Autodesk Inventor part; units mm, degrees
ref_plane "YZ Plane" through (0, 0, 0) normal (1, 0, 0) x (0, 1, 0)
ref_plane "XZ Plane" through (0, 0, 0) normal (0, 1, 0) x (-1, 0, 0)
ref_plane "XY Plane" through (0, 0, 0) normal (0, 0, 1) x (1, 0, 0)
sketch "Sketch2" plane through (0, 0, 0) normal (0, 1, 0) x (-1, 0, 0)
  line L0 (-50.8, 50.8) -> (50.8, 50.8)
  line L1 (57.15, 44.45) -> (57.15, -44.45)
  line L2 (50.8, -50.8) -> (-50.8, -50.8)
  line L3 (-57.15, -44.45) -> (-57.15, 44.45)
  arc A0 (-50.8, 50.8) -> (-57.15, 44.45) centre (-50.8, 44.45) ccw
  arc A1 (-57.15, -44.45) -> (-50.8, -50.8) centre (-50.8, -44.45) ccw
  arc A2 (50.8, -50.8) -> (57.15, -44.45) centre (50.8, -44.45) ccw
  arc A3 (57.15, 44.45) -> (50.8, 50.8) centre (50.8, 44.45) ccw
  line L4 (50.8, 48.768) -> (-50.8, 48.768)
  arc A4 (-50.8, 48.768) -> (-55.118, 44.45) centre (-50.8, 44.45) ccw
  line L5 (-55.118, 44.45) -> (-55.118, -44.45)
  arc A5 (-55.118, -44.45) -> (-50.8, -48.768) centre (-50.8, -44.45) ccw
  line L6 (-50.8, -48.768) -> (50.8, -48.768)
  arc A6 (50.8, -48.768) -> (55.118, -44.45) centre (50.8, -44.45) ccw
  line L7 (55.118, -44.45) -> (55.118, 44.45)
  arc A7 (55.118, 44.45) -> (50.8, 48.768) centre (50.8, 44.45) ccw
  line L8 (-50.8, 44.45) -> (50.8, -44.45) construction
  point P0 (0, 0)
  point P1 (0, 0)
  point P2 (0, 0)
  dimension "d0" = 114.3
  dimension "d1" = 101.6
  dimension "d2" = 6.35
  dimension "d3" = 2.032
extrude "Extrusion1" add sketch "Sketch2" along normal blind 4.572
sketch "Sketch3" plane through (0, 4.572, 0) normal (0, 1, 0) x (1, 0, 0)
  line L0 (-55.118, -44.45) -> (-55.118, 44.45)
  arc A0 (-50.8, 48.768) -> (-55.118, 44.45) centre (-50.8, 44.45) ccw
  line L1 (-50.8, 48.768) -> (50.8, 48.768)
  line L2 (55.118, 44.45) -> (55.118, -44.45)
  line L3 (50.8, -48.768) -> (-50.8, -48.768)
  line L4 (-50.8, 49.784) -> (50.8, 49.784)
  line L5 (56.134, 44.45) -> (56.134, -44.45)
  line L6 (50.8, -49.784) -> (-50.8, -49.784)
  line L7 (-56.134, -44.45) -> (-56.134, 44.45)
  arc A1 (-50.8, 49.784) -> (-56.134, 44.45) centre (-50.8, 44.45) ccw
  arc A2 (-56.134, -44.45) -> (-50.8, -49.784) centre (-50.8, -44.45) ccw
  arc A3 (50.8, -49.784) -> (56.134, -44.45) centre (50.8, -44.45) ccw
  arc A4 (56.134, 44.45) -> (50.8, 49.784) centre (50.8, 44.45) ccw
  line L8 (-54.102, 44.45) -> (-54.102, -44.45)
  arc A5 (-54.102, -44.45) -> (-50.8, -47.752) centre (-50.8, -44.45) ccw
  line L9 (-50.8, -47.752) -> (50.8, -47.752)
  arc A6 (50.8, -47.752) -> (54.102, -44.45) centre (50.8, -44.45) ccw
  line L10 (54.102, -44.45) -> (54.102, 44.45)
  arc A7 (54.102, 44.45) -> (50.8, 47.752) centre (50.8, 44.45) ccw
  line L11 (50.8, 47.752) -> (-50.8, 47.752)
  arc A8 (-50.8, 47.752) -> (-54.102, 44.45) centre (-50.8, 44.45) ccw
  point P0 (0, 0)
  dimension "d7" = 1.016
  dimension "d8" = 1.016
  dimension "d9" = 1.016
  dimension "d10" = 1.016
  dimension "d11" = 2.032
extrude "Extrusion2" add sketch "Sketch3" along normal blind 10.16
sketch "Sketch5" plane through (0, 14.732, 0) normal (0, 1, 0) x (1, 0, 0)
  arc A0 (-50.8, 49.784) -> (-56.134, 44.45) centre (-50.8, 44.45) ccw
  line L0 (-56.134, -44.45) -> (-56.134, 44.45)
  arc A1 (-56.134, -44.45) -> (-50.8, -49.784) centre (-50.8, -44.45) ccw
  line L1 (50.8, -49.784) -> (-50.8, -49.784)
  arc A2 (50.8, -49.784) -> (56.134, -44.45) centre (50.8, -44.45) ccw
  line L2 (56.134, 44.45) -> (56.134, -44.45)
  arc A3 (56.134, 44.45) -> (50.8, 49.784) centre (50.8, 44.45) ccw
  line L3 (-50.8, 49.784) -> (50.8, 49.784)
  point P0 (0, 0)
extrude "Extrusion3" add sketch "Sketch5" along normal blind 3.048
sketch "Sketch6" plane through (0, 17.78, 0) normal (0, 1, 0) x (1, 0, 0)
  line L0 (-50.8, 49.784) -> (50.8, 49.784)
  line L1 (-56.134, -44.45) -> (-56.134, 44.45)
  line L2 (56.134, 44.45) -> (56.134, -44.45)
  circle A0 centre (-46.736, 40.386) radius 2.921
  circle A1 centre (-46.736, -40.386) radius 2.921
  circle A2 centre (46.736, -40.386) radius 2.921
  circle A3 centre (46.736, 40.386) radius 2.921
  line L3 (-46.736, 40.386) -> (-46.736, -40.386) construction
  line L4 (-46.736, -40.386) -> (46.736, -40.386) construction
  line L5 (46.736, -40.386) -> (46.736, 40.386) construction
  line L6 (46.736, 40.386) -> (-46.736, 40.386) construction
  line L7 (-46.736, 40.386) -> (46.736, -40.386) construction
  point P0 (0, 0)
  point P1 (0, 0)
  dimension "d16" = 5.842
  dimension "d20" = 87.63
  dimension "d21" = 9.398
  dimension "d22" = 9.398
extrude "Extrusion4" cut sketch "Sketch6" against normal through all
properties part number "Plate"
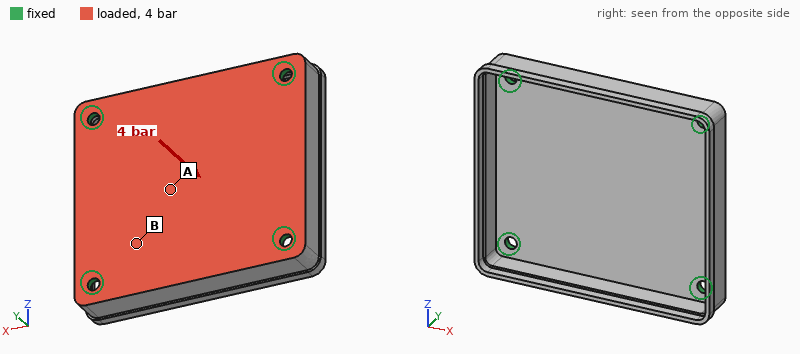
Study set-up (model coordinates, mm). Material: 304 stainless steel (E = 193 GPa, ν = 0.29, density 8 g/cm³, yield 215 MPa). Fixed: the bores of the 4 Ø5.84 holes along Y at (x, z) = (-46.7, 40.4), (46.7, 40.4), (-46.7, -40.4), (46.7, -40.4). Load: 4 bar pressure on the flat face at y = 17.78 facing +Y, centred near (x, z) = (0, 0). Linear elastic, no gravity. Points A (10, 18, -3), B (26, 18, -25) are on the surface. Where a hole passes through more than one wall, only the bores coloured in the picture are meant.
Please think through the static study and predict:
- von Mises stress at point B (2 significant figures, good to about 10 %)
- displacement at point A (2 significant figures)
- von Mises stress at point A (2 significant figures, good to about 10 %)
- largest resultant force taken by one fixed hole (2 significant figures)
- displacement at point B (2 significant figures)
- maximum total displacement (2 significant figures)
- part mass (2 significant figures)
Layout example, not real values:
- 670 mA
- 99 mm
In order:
- 44 MPa
- 0.23 mm
- 91 MPa
- 1.1 kN
- 0.11 mm
- 0.24 mm
- 370 g
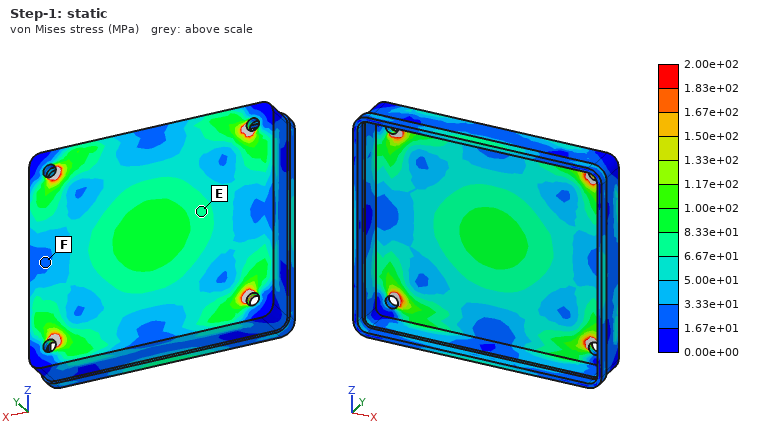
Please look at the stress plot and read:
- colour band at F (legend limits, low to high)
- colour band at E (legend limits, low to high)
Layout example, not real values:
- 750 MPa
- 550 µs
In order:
- 1.67e+01 to 3.33e+01 MPa
- 6.67e+01 to 8.33e+01 MPa
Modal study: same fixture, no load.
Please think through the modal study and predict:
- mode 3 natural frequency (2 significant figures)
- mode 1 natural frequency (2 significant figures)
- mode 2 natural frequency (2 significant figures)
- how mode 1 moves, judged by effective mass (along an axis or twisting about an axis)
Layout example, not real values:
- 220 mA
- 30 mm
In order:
- 3600 Hz
- 1600 Hz
- 3500 Hz
- along Y
